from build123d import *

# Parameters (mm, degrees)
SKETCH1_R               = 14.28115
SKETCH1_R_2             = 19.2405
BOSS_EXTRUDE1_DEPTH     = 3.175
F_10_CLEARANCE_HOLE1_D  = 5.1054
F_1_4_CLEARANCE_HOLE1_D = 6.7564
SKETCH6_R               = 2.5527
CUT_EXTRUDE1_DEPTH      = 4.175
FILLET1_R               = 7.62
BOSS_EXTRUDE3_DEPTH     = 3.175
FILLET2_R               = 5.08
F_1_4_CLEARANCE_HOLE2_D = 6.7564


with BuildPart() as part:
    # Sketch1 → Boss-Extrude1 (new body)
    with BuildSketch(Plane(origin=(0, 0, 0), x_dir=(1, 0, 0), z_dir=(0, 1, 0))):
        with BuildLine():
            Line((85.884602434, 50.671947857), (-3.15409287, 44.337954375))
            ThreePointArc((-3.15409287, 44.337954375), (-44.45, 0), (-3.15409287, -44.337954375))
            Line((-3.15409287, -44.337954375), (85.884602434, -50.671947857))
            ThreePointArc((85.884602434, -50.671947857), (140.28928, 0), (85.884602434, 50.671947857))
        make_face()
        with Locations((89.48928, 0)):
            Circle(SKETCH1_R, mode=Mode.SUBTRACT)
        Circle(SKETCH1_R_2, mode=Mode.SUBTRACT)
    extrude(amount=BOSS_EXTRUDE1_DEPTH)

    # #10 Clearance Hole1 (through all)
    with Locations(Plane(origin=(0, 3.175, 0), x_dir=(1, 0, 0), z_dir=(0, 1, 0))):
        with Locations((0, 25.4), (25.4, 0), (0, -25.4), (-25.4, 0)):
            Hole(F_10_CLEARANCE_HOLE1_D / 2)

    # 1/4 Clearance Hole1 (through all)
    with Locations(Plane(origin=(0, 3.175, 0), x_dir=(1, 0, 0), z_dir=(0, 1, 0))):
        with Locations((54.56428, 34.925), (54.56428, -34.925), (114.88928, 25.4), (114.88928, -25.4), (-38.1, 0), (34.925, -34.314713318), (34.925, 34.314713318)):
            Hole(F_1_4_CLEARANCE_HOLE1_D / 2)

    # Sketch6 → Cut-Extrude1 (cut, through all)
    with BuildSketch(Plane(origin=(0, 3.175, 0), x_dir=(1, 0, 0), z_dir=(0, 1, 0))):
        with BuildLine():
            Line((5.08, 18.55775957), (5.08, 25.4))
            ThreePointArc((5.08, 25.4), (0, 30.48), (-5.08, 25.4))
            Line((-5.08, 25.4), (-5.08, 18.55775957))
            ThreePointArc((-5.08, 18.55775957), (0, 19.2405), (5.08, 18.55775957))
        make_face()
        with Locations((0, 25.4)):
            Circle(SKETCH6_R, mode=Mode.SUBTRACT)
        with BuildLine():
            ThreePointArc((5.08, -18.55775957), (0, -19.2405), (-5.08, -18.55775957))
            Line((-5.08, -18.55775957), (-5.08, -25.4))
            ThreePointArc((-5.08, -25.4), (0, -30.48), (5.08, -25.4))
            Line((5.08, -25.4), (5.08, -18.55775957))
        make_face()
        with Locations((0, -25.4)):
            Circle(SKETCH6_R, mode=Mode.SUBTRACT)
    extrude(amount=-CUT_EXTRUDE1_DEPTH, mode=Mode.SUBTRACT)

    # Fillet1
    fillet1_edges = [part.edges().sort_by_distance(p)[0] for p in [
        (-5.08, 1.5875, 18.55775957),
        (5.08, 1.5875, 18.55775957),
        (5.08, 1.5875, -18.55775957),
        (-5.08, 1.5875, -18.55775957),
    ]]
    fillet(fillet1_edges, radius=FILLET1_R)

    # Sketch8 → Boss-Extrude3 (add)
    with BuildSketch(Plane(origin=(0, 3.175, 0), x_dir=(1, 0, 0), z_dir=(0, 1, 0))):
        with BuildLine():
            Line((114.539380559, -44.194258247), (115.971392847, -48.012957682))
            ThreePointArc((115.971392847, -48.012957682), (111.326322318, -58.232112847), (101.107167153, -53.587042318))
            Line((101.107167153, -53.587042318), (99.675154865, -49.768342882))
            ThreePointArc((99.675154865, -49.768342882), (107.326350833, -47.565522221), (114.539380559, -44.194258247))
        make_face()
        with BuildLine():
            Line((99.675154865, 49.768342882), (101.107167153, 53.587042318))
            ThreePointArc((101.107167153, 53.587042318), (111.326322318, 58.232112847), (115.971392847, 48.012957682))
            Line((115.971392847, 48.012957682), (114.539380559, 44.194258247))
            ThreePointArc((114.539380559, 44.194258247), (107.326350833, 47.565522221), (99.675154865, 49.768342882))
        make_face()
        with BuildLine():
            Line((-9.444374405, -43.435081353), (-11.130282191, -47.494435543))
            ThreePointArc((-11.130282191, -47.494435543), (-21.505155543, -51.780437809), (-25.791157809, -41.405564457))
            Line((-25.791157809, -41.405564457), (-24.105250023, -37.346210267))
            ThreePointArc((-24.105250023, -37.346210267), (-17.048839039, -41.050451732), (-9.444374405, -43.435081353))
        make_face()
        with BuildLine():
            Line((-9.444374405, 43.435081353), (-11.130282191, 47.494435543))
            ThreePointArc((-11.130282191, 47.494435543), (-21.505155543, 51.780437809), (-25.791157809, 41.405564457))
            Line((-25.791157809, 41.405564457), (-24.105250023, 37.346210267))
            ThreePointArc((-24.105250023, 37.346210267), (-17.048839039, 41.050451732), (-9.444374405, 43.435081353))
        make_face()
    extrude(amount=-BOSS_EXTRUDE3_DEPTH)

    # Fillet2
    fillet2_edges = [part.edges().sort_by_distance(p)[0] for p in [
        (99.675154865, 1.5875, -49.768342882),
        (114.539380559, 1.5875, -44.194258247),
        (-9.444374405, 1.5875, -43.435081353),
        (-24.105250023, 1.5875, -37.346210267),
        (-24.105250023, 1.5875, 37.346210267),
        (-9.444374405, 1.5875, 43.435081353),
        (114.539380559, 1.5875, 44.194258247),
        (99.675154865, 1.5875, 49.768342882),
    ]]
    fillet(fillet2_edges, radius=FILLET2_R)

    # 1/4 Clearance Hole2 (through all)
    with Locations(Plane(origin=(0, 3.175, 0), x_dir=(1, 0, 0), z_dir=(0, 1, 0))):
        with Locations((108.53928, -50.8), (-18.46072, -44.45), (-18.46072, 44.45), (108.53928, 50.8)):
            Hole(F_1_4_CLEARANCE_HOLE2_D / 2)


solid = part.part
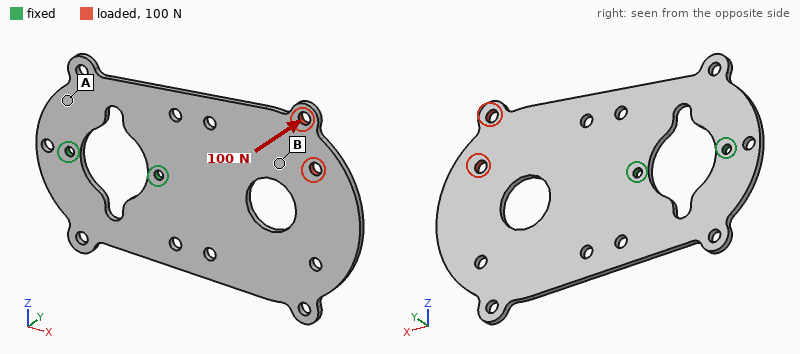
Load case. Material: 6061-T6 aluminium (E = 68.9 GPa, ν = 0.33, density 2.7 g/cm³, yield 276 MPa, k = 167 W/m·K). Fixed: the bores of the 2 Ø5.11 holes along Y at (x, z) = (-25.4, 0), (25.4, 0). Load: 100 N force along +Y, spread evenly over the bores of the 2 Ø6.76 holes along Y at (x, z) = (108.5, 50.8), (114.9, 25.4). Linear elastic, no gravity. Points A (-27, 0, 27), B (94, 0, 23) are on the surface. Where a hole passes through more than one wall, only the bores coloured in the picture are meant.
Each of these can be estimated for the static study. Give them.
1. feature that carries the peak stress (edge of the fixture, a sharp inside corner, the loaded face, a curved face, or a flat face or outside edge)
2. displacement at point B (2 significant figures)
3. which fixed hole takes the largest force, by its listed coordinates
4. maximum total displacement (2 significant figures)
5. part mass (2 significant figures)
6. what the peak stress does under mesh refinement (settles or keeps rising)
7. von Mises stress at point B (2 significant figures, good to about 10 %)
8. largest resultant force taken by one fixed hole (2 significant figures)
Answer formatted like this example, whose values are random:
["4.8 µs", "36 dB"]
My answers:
["edge of the fixture", "1.4 mm", "(25.4, 0)", "2.6 mm", "120 g", "keeps rising", "17 MPa", "160 N"]
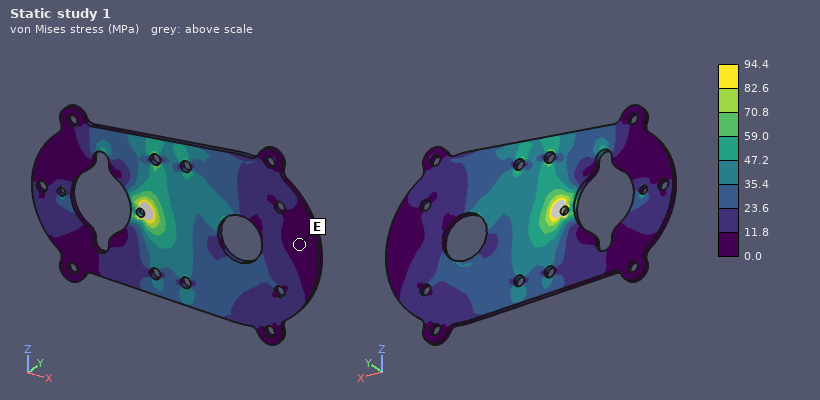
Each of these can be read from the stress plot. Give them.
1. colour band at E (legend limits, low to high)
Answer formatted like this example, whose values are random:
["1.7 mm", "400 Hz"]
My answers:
["0.0 to 11.8 MPa"]
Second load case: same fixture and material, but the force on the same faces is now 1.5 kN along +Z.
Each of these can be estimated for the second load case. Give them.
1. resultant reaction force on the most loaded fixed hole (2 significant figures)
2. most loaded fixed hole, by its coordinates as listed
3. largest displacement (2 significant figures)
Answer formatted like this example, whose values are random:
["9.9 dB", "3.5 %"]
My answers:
["3.6 kN", "(25.4, 0)", "0.26 mm"]
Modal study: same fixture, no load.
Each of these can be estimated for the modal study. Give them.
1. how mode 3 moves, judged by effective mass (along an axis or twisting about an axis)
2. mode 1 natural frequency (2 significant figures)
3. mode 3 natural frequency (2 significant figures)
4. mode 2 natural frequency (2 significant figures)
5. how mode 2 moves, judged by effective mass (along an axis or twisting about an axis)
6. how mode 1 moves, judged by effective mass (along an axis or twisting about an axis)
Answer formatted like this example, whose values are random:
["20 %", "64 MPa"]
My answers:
["along Y", "200 Hz", "940 Hz", "390 Hz", "twisting about X", "along Y"]
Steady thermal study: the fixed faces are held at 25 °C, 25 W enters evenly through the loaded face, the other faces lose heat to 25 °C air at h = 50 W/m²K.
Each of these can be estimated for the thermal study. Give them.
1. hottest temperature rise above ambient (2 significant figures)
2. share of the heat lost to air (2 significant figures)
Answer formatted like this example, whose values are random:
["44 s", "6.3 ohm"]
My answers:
["54 K", "71 %"]
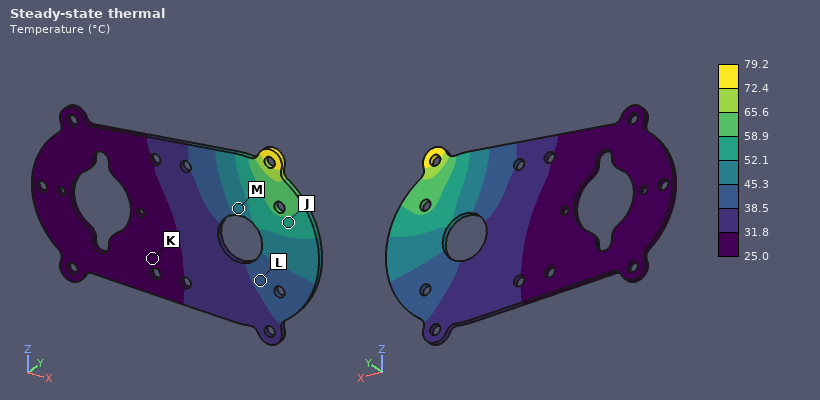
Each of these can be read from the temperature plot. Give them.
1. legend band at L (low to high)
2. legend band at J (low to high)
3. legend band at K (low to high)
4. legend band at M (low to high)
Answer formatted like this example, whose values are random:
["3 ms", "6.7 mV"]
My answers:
["38.5 to 45.3 °C", "52.1 to 58.9 °C", "25.0 to 31.8 °C", "45.3 to 52.1 °C"]
